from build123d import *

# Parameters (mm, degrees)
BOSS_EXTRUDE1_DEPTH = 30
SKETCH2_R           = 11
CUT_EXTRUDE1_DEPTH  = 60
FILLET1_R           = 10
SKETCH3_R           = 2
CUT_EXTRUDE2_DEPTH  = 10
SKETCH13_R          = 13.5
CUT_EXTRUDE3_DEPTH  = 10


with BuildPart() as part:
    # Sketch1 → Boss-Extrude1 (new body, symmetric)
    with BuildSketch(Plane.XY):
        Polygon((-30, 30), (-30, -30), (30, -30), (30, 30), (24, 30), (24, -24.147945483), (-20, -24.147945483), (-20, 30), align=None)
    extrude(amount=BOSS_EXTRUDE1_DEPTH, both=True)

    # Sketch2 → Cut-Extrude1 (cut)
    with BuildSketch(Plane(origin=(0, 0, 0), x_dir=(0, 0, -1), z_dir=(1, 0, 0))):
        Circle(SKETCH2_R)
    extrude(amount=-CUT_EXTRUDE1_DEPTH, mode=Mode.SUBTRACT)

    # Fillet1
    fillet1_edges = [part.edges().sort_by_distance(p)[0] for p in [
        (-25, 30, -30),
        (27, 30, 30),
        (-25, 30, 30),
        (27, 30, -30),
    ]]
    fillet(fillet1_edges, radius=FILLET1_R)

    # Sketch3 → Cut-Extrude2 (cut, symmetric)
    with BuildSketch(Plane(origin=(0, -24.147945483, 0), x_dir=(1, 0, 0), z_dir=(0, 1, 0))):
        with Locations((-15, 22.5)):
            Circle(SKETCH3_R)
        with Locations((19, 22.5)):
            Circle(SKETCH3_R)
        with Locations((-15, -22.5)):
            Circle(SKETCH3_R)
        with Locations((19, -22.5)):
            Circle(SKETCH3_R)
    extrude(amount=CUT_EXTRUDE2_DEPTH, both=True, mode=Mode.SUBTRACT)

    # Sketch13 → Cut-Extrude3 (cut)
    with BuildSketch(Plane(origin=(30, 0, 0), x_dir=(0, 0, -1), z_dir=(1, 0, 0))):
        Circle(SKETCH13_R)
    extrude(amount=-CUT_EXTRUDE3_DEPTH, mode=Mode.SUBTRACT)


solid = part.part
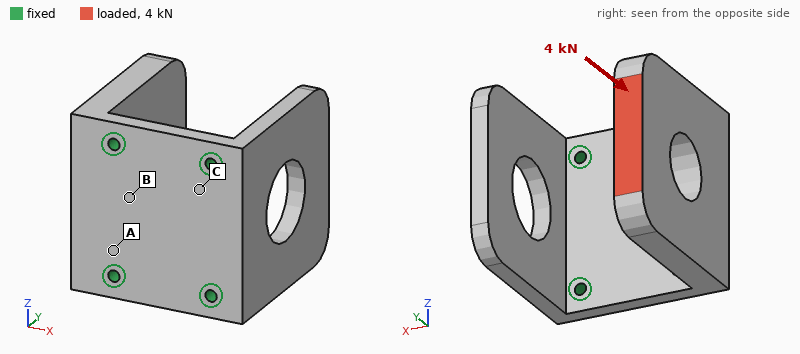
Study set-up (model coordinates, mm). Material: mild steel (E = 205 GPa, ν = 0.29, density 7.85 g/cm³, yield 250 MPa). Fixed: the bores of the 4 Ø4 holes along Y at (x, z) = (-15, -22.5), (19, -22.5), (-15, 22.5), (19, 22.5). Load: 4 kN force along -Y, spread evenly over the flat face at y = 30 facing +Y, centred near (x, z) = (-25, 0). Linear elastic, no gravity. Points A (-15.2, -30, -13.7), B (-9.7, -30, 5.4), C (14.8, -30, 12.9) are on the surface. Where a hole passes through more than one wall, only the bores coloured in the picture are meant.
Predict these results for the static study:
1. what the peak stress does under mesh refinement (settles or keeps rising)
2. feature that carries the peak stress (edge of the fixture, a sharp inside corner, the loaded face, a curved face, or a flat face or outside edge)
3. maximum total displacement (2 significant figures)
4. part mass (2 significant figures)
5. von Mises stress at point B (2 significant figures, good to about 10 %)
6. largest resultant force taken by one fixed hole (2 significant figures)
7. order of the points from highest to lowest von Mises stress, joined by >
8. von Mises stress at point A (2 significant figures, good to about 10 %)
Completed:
keeps rising
edge of the fixture
74 µm
510 g
26 MPa
2.2 kN
A > B > C
45 MPa
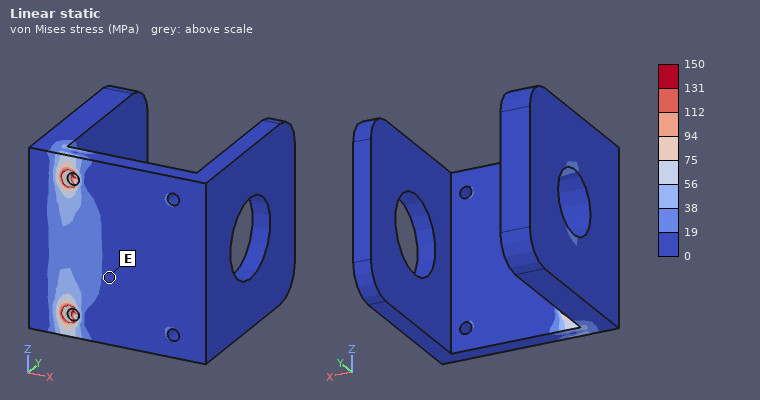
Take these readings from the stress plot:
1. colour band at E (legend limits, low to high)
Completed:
0 to 19 MPa
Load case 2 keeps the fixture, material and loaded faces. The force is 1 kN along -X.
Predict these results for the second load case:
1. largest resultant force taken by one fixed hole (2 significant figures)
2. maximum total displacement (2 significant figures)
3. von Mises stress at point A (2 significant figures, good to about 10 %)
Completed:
460 N
0.22 mm
86 MPa
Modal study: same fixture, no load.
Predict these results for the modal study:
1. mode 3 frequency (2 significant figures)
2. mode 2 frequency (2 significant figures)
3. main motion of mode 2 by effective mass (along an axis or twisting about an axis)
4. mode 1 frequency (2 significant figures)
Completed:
3000 Hz
1300 Hz
along X
1200 Hz
